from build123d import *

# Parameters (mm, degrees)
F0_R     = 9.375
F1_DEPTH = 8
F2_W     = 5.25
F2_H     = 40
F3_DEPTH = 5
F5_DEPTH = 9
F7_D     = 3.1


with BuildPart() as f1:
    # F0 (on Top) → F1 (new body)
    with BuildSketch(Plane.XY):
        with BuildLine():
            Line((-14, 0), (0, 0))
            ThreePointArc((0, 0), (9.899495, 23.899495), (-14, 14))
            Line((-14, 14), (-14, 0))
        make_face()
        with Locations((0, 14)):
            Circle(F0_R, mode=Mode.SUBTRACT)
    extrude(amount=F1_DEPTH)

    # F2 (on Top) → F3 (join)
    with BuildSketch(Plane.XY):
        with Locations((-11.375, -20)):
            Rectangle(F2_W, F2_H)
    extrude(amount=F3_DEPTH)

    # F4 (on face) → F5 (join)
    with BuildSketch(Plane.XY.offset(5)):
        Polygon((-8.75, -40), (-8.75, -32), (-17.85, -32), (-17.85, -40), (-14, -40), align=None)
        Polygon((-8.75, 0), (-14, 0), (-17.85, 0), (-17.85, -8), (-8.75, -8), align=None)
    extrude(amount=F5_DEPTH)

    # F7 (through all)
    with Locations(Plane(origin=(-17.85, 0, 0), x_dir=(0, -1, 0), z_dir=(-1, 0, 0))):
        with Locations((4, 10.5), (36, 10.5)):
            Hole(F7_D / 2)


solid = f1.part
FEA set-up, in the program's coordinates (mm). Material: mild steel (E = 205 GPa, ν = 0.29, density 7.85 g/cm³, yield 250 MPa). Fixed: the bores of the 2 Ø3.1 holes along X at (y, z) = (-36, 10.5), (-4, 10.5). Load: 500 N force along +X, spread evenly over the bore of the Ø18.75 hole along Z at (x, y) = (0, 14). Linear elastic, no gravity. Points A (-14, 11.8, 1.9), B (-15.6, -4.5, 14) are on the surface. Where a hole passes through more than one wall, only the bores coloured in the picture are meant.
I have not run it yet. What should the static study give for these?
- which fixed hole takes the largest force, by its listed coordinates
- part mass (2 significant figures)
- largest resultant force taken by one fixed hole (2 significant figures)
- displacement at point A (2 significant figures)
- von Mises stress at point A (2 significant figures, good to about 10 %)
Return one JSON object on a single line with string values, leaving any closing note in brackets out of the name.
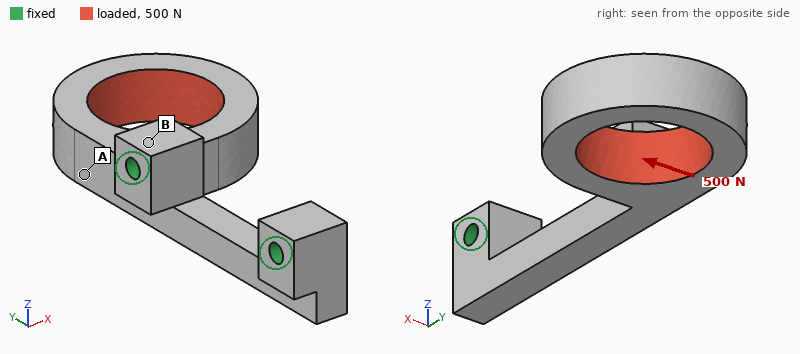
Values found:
{"which fixed hole takes the largest force, by its listed coordinates": "(-4, 10.5)", "part mass": "41 g", "largest resultant force taken by one fixed hole": "550 N", "displacement at point A": "35 µm", "von Mises stress at point A": "41 MPa"}
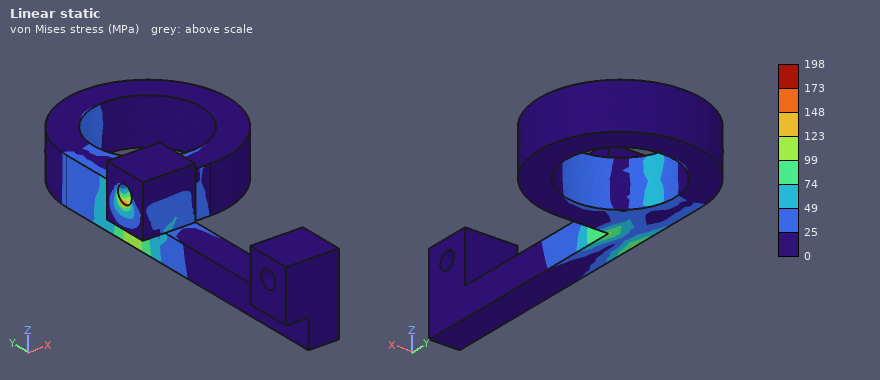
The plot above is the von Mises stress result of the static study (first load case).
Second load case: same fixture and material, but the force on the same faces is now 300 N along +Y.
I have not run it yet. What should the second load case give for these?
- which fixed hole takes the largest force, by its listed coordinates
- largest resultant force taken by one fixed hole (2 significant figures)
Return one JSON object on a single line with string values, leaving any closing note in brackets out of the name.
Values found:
{"which fixed hole takes the largest force, by its listed coordinates": "(-4, 10.5)", "largest resultant force taken by one fixed hole": "210 N"}
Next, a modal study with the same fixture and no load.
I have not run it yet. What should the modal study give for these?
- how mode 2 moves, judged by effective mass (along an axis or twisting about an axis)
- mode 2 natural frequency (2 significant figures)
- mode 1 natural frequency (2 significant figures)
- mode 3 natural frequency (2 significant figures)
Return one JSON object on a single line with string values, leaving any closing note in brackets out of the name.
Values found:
{"how mode 2 moves, judged by effective mass": "along Z", "mode 2 natural frequency": "2900 Hz", "mode 1 natural frequency": "2500 Hz", "mode 3 natural frequency": "6300 Hz"}
